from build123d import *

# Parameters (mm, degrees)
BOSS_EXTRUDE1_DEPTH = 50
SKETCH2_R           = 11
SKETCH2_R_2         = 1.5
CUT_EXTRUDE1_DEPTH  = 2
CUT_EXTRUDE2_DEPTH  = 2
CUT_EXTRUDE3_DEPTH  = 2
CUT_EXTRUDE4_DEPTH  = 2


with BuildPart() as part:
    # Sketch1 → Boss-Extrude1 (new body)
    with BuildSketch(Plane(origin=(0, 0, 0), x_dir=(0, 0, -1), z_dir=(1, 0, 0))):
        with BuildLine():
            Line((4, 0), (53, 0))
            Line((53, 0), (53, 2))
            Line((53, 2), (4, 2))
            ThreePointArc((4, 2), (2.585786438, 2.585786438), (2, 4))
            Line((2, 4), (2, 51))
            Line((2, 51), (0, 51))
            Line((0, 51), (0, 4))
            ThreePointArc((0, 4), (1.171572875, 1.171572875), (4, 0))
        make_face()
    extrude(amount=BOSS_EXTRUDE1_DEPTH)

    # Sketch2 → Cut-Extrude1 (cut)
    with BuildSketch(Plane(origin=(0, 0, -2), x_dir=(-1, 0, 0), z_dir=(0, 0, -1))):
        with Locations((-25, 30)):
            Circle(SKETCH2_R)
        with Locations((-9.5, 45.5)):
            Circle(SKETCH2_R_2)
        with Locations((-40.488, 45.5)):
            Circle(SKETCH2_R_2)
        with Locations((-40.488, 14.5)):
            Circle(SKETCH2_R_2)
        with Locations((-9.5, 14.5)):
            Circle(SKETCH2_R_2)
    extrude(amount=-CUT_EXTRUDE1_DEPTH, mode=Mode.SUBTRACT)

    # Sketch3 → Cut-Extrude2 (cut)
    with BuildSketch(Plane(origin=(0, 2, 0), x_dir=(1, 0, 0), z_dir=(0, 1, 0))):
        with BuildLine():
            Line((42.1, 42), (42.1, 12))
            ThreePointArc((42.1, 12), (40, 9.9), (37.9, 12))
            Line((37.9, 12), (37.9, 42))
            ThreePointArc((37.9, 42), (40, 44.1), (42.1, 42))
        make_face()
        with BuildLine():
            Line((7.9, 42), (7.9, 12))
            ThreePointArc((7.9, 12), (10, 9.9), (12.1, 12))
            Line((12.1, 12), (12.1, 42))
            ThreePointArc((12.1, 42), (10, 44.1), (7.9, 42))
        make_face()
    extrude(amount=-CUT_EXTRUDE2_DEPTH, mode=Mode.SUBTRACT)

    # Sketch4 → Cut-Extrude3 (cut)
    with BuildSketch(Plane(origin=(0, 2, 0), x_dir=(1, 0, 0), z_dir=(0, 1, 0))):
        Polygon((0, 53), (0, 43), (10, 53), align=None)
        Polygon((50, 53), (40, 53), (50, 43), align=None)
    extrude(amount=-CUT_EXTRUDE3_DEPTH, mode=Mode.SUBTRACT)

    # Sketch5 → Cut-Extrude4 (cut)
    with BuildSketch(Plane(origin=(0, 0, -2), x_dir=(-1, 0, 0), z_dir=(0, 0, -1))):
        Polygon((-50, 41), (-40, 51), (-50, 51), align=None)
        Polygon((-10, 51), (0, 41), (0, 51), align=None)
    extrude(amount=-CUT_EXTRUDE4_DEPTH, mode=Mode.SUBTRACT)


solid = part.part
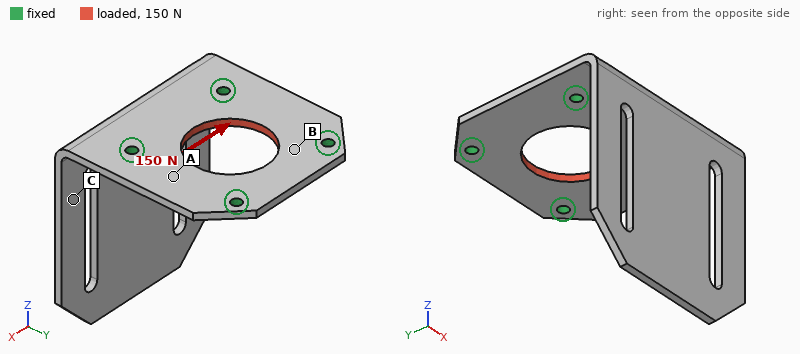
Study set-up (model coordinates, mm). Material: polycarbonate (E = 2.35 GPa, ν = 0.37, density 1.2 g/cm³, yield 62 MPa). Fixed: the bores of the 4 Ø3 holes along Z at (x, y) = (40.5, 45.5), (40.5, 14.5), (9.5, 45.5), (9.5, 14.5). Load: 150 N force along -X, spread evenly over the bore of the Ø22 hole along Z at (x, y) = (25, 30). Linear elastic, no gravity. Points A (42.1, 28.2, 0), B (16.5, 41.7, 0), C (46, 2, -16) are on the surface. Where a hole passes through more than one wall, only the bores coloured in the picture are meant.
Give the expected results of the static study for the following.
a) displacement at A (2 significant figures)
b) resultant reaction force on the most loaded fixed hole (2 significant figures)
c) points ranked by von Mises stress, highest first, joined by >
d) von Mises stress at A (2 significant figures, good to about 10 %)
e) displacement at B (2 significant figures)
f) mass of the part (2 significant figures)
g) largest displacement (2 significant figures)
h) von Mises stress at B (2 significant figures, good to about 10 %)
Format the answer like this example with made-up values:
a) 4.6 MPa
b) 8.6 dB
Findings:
a) 14 µm
b) 39 N
c) B > A > C
d) 0.80 MPa
e) 6.9 µm
f) 10.0 g
g) 16 µm
h) 1.5 MPa
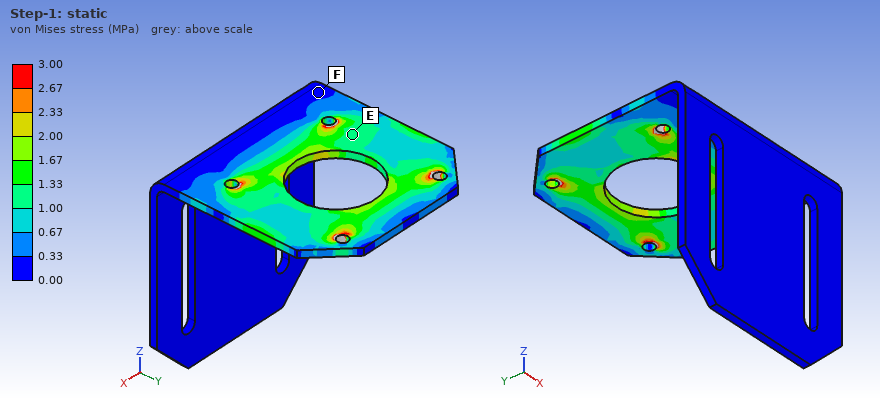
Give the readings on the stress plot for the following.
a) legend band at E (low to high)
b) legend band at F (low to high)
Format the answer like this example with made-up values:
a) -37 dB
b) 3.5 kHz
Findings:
a) 1.00 to 1.33 MPa
b) 0.00 to 0.33 MPa
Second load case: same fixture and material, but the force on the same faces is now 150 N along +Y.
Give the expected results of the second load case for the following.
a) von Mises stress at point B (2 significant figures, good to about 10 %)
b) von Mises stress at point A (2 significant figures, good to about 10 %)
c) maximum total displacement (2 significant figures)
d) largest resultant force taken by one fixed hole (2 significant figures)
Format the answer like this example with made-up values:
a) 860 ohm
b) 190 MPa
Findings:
a) 1.5 MPa
b) 0.86 MPa
c) 22 µm
d) 40 N
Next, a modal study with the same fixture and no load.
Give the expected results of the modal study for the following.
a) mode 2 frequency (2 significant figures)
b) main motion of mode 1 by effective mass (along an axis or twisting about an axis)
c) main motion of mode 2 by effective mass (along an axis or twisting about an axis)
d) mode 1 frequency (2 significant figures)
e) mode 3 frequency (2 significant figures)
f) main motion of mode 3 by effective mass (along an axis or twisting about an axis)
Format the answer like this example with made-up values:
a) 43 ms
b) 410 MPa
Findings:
a) 350 Hz
b) along Y
c) along X
d) 130 Hz
e) 520 Hz
f) along X
